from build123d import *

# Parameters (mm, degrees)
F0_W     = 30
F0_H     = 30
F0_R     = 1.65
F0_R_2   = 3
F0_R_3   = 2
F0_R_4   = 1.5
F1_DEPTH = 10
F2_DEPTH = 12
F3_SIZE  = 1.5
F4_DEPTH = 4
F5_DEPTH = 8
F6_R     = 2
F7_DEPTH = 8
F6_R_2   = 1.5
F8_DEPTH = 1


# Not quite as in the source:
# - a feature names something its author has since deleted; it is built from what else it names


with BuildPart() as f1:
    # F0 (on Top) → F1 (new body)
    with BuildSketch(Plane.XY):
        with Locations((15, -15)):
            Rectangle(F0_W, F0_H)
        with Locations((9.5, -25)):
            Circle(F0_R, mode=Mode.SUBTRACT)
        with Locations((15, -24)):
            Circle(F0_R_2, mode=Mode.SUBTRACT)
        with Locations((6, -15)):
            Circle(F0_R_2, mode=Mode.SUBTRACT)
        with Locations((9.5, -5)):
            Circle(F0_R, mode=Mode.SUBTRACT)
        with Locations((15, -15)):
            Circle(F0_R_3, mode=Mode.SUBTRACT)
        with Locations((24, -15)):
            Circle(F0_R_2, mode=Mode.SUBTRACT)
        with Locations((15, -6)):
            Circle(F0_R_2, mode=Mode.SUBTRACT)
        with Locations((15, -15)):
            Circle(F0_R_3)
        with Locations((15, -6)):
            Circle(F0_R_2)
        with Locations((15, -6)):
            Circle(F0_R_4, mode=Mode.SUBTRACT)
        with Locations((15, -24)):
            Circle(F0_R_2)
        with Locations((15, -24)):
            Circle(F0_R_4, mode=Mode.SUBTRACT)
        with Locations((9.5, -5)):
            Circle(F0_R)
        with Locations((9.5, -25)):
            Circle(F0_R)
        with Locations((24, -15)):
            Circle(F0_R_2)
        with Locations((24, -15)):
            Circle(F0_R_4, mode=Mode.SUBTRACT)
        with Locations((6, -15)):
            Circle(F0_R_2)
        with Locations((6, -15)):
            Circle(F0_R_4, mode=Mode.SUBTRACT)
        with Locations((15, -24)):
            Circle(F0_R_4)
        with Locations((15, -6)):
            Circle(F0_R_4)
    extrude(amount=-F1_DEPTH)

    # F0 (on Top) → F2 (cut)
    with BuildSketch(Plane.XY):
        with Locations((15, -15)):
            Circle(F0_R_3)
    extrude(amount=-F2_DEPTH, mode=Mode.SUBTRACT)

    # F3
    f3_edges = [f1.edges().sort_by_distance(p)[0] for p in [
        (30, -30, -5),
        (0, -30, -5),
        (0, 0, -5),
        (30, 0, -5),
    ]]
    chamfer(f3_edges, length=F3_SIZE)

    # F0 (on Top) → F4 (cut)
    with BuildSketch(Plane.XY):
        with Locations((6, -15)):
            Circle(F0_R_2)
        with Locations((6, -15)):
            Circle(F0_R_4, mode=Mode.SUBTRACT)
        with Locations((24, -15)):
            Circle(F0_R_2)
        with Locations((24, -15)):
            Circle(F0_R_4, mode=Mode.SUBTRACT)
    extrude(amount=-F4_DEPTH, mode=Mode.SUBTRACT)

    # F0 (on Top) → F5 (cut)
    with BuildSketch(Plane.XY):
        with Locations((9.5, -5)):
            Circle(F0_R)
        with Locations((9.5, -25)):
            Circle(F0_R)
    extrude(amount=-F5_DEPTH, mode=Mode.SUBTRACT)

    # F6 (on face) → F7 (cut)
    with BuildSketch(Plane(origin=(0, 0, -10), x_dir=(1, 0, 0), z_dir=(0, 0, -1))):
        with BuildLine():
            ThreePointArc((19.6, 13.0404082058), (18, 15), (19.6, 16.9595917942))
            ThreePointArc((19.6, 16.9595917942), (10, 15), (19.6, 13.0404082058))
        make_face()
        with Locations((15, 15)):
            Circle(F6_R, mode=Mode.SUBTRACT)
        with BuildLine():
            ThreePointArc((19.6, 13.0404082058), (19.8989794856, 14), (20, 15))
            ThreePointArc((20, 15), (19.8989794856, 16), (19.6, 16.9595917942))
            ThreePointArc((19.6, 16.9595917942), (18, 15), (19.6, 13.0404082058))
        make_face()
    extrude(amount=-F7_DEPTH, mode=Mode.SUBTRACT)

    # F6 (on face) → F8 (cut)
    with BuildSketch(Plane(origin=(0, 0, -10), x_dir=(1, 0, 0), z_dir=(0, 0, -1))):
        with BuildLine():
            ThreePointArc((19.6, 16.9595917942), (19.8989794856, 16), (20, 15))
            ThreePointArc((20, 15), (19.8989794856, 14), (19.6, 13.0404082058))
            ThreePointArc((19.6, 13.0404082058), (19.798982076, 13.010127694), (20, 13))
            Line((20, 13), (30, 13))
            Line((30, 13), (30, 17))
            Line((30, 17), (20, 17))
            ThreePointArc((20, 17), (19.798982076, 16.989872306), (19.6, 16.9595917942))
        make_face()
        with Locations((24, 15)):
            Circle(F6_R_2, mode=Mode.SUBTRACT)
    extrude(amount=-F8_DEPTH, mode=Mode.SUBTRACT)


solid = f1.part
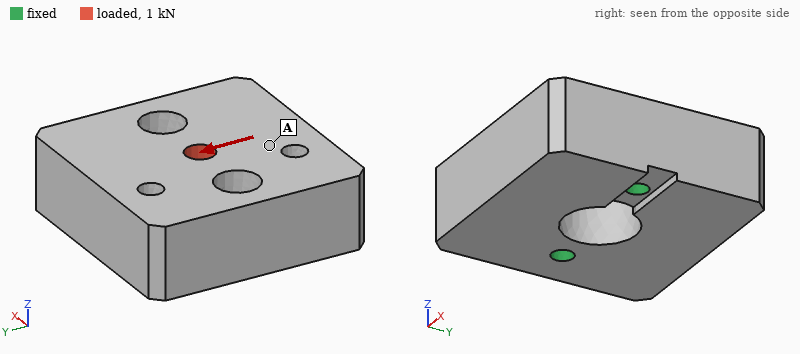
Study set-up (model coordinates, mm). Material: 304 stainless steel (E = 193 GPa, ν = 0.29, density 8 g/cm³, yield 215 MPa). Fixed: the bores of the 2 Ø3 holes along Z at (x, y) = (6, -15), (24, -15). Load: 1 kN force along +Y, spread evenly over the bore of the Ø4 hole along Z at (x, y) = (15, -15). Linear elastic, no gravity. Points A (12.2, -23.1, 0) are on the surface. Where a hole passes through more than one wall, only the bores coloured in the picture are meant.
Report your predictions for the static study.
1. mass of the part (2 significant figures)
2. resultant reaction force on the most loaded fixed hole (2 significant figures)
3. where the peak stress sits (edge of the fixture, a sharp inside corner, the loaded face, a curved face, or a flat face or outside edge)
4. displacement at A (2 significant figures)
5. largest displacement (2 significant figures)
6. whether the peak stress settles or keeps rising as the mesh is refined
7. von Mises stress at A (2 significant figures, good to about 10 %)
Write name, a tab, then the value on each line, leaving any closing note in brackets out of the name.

mass of the part	63 g
resultant reaction force on the most loaded fixed hole	500 N
where the peak stress sits	edge of the fixture
displacement at A	2.4 µm
largest displacement	3.6 µm
whether the peak stress settles or keeps rising as the mesh is refined	keeps rising
von Mises stress at A	10 MPa
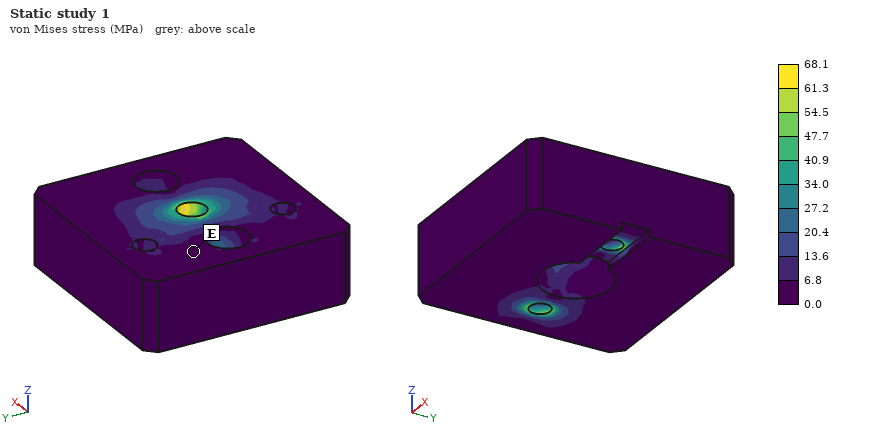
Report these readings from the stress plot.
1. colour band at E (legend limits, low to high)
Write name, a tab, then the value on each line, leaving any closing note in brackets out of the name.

colour band at E	0.0 to 6.8 MPa
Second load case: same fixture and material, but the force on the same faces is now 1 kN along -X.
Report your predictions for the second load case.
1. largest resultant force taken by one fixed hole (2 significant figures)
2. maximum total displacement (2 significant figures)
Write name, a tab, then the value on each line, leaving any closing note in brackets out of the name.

largest resultant force taken by one fixed hole	560 N
maximum total displacement	1.8 µm
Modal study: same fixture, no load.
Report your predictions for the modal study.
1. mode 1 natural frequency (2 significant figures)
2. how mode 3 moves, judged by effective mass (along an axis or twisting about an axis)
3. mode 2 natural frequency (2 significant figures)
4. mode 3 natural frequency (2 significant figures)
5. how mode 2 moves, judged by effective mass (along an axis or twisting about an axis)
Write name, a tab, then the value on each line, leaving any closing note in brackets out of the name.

mode 1 natural frequency	11 kHz
how mode 3 moves, judged by effective mass	twisting about Z
mode 2 natural frequency	21 kHz
mode 3 natural frequency	24 kHz
how mode 2 moves, judged by effective mass	along Z
